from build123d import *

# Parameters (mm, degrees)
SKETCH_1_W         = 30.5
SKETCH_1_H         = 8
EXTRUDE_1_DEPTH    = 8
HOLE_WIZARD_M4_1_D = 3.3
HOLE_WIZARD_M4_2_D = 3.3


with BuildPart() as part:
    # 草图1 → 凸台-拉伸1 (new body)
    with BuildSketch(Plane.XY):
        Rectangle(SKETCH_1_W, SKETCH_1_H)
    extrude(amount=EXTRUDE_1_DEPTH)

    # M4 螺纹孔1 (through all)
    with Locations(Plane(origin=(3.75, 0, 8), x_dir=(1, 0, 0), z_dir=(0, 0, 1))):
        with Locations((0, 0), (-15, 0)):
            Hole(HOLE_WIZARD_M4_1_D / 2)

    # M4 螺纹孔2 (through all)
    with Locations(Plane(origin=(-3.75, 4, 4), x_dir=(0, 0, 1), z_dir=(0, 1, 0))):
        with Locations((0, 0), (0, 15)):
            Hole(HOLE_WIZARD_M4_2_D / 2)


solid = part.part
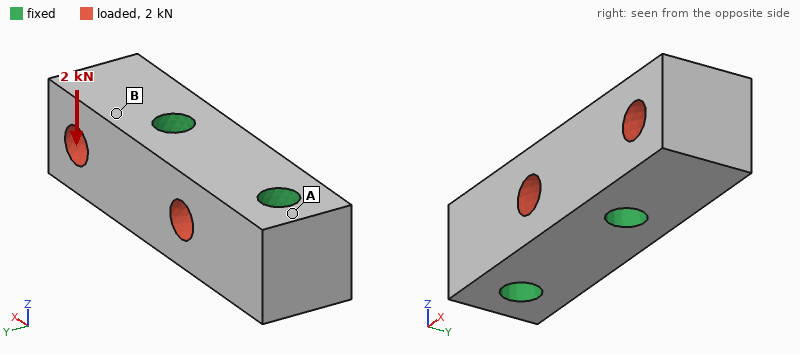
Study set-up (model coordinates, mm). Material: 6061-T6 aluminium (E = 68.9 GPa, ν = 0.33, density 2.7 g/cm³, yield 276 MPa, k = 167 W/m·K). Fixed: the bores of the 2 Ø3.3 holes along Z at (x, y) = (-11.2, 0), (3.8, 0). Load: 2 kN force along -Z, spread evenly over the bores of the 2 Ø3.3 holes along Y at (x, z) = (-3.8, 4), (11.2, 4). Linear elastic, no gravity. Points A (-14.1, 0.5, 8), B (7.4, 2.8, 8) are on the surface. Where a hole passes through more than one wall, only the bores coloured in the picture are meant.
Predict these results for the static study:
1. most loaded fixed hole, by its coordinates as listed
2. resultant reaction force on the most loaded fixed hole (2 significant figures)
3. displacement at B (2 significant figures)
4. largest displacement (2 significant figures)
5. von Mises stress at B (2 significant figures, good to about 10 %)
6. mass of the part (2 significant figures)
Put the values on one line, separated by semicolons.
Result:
(3.8, 0); 1.5 kN; 4.7 µm; 17 µm; 45 MPa; 4.5 g
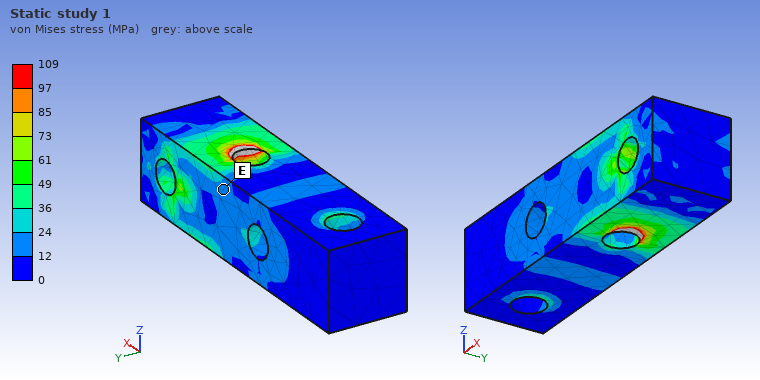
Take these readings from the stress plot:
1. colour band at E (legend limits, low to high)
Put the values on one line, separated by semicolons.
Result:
12 to 24 MPa
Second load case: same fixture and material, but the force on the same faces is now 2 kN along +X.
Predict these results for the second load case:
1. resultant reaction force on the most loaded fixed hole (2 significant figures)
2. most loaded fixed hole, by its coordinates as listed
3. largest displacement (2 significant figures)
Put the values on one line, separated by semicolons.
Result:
1.5 kN; (3.8, 0); 3.0 µm
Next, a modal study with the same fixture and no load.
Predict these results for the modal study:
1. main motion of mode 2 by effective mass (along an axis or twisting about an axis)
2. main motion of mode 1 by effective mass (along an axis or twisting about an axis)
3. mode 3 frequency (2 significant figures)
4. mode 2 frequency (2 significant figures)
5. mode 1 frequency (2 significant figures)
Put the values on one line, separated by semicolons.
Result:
along Z; along Y; 63 kHz; 40 kHz; 35 kHz
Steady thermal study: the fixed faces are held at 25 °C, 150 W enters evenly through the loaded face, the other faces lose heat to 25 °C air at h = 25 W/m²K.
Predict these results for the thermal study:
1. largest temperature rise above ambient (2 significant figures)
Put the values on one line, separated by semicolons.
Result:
62 K
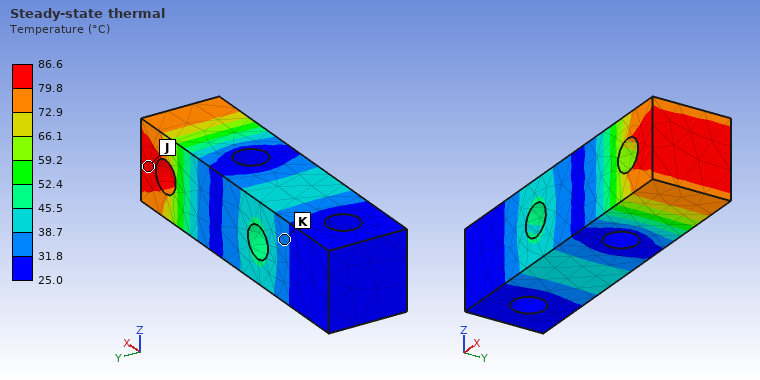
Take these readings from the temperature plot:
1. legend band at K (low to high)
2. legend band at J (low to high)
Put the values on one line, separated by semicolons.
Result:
31.8 to 38.7 °C; 79.8 to 86.6 °C
